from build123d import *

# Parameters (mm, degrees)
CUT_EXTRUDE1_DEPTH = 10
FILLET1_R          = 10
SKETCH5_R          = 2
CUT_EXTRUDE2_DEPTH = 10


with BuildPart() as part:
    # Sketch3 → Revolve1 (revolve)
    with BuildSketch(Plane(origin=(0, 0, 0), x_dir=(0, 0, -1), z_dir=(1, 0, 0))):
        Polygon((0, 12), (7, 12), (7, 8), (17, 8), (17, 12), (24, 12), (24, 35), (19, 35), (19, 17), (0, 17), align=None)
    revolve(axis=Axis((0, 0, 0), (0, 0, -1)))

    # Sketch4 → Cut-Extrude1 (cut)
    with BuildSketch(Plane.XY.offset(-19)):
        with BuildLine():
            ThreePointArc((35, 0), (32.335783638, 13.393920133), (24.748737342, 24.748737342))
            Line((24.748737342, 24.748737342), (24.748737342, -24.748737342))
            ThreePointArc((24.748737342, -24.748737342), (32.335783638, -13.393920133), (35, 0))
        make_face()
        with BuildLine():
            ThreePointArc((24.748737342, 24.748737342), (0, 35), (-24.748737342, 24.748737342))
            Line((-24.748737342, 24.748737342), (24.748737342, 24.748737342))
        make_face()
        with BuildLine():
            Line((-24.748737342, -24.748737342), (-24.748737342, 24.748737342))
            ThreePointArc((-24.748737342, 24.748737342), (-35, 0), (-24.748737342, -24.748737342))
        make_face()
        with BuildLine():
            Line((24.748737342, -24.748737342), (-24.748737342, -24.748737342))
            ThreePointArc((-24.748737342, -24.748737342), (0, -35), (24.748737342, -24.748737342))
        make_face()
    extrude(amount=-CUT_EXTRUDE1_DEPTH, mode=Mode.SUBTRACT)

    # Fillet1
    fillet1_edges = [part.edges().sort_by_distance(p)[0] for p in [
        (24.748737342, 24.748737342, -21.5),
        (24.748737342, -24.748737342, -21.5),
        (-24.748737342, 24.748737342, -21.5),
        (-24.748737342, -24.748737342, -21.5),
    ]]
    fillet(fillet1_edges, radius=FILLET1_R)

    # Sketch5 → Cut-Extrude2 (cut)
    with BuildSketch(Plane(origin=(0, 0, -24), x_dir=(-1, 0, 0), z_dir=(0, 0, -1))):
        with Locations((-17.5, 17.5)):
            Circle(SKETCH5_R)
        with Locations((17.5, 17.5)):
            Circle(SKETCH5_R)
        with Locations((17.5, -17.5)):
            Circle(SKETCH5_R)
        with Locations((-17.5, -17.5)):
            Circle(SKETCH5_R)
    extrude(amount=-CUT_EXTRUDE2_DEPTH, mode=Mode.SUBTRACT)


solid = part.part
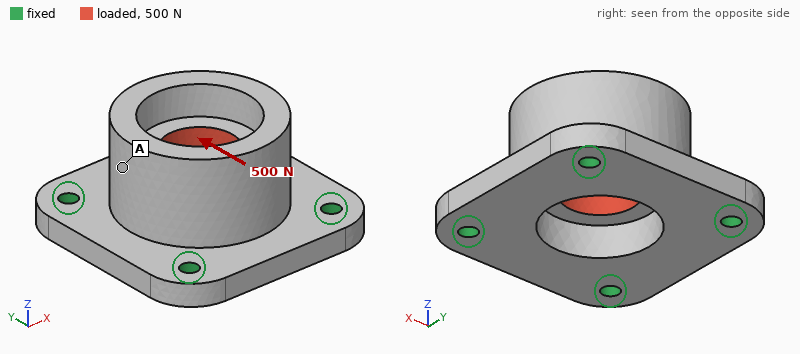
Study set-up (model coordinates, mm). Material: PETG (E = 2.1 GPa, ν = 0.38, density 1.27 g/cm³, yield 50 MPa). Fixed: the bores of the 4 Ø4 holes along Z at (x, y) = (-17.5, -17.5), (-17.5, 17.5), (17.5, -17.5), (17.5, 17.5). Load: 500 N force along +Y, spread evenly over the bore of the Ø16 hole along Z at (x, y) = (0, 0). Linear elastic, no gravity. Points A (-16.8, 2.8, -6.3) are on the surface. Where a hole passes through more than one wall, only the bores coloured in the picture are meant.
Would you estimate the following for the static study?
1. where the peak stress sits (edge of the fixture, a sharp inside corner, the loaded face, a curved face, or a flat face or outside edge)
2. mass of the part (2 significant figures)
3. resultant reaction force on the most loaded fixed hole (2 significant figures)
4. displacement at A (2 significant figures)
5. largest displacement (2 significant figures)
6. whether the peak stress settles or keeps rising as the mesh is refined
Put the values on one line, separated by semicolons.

edge of the fixture; 26 g; 150 N; 50 µm; 72 µm; keeps rising
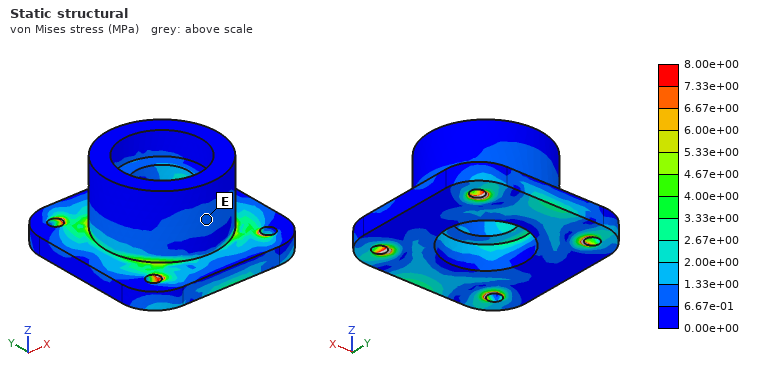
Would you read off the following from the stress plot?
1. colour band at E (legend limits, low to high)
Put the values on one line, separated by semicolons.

6.67e-01 to 1.33e+00 MPa
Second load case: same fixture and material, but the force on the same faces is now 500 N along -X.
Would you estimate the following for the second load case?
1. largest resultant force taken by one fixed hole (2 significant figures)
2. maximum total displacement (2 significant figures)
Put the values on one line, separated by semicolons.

150 N; 72 µm
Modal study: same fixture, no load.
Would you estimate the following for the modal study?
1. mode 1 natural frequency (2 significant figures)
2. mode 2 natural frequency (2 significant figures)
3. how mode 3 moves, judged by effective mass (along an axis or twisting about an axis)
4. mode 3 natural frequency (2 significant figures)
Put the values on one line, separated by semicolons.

3200 Hz; 3200 Hz; along Z; 3400 Hz
